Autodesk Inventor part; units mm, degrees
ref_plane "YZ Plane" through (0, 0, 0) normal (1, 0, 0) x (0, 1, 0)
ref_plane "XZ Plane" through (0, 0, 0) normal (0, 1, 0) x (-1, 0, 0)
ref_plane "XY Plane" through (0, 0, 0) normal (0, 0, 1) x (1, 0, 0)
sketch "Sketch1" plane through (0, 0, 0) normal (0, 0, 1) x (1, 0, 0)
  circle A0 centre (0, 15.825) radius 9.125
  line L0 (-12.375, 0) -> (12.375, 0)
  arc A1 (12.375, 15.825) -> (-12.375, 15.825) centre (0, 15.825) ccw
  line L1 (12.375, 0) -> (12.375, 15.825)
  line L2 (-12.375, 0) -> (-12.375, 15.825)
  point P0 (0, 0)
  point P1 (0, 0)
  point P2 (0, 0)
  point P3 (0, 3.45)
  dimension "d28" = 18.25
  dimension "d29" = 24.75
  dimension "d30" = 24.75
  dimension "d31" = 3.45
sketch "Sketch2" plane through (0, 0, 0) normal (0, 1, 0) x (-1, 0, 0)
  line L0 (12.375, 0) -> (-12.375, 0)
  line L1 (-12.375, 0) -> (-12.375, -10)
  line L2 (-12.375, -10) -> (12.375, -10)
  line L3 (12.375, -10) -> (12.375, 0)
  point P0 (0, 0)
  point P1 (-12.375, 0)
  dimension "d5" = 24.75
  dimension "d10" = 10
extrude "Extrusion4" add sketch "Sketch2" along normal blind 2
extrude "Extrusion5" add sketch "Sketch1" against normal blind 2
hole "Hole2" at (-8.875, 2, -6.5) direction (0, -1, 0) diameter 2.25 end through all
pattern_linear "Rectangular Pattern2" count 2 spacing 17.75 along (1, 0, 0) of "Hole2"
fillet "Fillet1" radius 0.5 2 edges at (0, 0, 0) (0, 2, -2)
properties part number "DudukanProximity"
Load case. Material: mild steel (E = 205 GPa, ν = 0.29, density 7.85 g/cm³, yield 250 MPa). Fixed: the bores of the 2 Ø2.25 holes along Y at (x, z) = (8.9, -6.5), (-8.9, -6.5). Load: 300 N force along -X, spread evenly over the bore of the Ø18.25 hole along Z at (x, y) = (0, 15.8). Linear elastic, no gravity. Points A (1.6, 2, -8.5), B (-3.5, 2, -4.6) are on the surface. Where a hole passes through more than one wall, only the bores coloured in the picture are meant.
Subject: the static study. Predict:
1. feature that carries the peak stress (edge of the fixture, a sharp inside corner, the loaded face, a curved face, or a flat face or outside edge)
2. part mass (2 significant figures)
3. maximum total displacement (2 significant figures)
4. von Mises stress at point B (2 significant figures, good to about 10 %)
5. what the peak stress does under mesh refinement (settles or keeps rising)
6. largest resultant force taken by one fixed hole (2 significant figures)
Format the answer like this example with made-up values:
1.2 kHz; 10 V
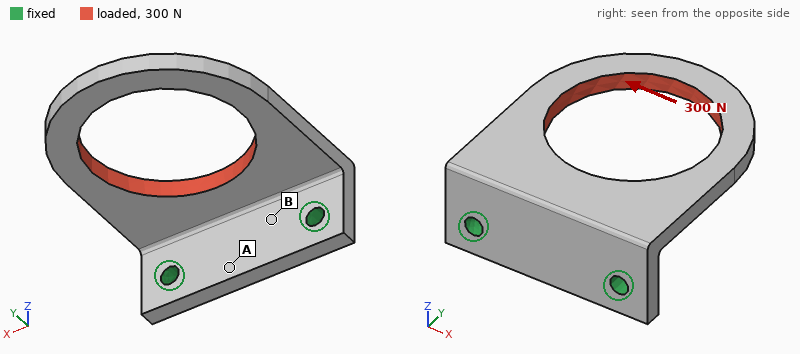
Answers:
edge of the fixture; 8.8 g; 42 µm; 42 MPa; keeps rising; 290 N
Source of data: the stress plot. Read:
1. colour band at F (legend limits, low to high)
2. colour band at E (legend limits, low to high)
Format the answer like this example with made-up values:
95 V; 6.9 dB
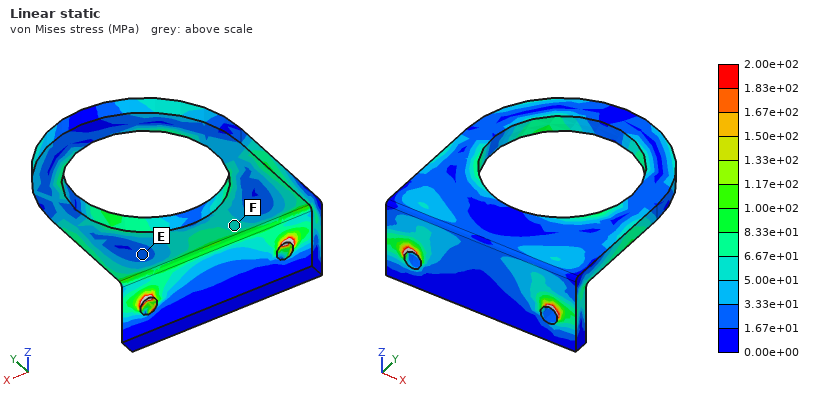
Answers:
5.00e+01 to 6.67e+01 MPa; 1.67e+01 to 3.33e+01 MPa
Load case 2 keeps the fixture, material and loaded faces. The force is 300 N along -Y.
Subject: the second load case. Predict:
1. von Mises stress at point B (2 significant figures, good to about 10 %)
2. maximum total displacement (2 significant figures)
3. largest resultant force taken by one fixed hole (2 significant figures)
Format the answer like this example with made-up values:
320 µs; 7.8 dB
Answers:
29 MPa; 42 µm; 150 N
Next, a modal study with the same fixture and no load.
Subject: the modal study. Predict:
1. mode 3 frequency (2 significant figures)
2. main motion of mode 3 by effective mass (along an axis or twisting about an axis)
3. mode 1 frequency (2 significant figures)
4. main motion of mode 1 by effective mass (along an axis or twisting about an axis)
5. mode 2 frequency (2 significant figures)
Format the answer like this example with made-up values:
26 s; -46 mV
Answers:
8400 Hz; along X; 2200 Hz; along Z; 5600 Hz
